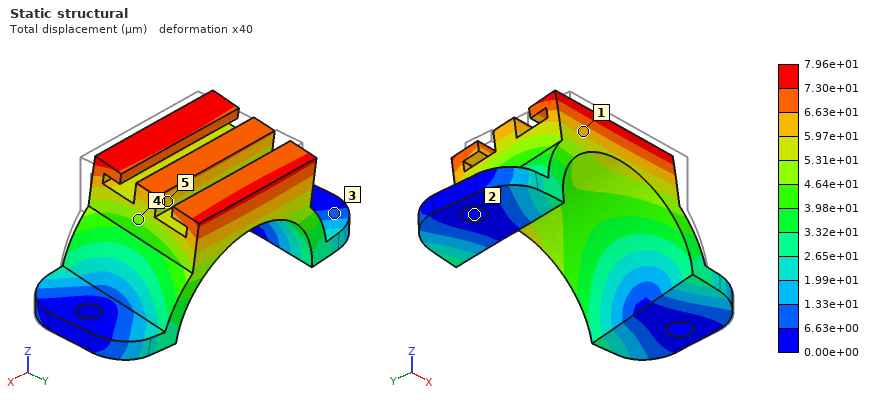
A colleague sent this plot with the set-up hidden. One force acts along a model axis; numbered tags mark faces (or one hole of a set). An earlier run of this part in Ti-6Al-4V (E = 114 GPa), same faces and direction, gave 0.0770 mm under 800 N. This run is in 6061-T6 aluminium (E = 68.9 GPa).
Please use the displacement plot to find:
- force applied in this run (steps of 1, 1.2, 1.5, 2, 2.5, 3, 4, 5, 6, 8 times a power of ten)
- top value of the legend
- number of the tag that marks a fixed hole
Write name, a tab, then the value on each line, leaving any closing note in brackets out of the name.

force applied in this run	500 N
top value of the legend	7.96e+01 µm
number of the tag that marks a fixed hole	2
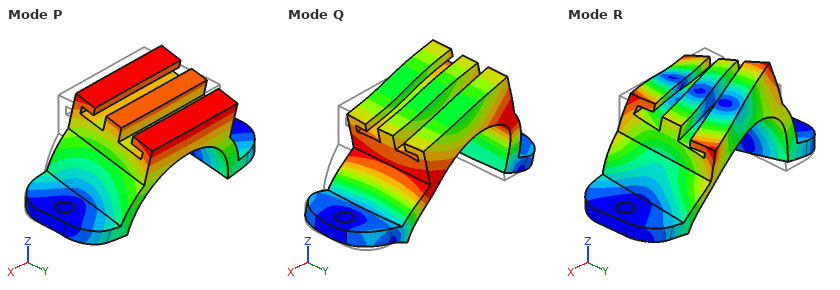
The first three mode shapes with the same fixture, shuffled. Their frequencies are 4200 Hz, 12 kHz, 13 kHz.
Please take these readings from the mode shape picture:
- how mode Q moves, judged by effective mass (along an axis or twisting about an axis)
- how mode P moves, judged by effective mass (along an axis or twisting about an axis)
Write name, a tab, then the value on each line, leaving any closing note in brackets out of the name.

how mode Q moves, judged by effective mass	along X
how mode P moves, judged by effective mass	along Y
